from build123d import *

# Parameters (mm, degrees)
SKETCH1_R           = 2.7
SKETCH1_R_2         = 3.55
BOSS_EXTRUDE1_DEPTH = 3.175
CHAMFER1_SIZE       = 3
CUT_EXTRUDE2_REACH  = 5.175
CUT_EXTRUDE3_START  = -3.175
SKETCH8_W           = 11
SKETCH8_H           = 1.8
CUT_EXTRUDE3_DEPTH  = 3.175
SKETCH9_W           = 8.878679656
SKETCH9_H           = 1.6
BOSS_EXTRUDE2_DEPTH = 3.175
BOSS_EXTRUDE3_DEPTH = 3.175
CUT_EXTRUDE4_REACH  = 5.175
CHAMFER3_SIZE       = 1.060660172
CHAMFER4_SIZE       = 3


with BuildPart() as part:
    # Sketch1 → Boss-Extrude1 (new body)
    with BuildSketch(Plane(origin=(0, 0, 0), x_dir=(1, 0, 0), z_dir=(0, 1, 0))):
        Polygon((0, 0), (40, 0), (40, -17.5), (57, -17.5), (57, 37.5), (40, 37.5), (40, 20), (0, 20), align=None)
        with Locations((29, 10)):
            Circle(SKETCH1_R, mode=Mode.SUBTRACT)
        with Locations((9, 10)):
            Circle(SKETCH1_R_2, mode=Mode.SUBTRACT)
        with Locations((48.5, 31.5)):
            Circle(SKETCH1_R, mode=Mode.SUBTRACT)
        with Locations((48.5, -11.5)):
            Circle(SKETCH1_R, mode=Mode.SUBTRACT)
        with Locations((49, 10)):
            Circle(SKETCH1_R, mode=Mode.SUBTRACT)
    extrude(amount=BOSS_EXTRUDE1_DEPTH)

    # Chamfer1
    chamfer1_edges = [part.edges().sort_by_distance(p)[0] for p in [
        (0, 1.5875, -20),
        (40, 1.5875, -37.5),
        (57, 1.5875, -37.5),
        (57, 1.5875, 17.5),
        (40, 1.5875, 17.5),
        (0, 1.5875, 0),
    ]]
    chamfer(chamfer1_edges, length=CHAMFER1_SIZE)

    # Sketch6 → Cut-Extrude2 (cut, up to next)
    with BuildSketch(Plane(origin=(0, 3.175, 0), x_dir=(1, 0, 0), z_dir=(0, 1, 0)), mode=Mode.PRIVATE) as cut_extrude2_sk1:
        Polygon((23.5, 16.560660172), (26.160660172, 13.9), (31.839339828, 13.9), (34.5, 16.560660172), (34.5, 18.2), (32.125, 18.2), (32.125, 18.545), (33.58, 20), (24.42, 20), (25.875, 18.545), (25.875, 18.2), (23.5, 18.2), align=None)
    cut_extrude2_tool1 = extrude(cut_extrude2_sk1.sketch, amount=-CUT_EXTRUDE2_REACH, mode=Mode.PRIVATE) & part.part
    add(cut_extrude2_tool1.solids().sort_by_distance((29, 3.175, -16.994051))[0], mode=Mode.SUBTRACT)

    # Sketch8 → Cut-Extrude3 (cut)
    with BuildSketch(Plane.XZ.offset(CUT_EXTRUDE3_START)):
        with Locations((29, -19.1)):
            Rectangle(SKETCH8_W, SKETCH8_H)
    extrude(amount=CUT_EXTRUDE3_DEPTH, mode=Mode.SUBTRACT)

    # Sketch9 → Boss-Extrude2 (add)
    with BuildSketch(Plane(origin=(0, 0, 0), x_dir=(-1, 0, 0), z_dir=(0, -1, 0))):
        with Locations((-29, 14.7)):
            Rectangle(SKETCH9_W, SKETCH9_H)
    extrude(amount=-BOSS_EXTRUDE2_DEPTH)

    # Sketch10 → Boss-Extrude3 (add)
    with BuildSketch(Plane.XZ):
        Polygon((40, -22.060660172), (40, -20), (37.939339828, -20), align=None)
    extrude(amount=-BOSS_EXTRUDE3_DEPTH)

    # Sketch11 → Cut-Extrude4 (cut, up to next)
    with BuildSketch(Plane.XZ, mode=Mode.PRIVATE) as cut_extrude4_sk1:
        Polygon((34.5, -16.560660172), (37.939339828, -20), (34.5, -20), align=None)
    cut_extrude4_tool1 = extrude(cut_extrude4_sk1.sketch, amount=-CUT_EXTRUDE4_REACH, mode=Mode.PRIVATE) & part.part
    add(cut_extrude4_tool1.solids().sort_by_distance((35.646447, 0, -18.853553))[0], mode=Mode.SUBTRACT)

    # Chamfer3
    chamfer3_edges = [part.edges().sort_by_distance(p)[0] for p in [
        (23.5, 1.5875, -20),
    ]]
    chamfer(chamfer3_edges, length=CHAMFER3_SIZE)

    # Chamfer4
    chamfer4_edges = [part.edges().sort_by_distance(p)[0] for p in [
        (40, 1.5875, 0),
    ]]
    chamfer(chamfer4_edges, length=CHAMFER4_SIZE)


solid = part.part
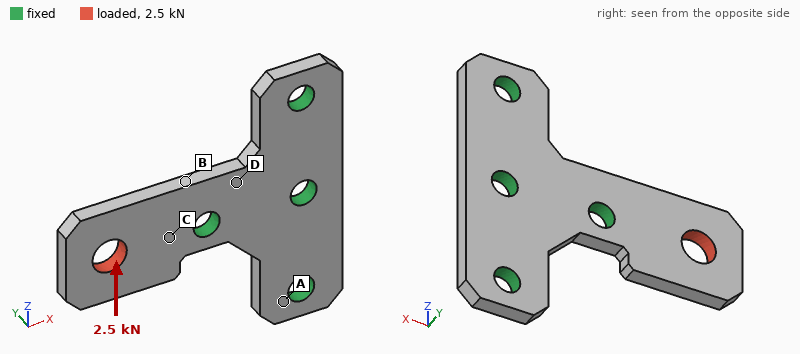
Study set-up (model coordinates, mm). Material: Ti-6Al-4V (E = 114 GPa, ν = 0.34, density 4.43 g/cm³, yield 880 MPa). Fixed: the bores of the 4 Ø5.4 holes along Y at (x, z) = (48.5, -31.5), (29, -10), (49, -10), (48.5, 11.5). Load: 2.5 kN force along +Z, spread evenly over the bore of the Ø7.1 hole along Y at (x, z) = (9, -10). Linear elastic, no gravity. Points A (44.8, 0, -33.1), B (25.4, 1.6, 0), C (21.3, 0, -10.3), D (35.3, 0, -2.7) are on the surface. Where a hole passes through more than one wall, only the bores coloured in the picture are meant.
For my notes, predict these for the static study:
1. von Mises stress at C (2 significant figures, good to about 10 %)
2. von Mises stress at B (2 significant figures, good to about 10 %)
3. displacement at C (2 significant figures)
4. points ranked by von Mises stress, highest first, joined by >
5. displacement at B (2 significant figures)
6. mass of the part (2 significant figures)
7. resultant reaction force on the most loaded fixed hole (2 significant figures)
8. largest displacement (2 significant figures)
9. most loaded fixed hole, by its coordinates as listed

170 MPa
280 MPa
0.030 mm
B > C > D > A
0.033 mm
21 g
3.7 kN
0.17 mm
(29, -10)
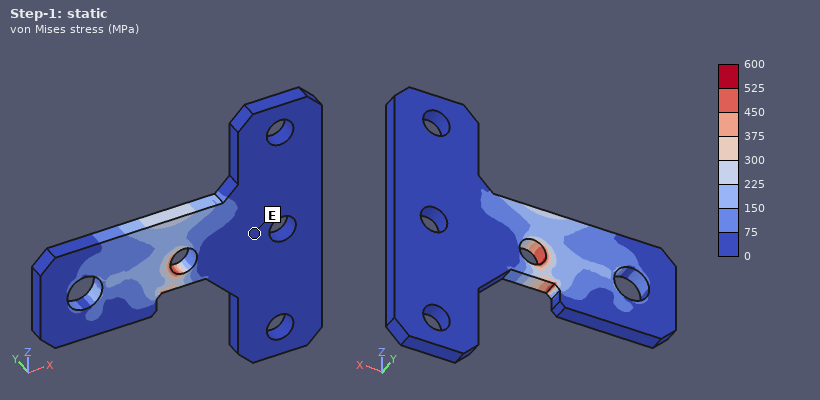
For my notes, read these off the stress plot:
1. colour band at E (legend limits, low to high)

0 to 75 MPa
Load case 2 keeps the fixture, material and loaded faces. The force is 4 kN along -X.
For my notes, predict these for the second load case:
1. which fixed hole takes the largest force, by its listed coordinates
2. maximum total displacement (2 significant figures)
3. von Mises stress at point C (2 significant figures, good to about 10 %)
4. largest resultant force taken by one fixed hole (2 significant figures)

(29, -10)
25 µm
100 MPa
3.7 kN
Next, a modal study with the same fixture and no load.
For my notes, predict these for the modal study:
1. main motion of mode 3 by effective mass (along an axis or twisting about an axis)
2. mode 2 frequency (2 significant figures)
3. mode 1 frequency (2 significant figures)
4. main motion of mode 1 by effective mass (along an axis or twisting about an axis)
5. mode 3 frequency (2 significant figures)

along Z
8300 Hz
3400 Hz
along Y
10 kHz
